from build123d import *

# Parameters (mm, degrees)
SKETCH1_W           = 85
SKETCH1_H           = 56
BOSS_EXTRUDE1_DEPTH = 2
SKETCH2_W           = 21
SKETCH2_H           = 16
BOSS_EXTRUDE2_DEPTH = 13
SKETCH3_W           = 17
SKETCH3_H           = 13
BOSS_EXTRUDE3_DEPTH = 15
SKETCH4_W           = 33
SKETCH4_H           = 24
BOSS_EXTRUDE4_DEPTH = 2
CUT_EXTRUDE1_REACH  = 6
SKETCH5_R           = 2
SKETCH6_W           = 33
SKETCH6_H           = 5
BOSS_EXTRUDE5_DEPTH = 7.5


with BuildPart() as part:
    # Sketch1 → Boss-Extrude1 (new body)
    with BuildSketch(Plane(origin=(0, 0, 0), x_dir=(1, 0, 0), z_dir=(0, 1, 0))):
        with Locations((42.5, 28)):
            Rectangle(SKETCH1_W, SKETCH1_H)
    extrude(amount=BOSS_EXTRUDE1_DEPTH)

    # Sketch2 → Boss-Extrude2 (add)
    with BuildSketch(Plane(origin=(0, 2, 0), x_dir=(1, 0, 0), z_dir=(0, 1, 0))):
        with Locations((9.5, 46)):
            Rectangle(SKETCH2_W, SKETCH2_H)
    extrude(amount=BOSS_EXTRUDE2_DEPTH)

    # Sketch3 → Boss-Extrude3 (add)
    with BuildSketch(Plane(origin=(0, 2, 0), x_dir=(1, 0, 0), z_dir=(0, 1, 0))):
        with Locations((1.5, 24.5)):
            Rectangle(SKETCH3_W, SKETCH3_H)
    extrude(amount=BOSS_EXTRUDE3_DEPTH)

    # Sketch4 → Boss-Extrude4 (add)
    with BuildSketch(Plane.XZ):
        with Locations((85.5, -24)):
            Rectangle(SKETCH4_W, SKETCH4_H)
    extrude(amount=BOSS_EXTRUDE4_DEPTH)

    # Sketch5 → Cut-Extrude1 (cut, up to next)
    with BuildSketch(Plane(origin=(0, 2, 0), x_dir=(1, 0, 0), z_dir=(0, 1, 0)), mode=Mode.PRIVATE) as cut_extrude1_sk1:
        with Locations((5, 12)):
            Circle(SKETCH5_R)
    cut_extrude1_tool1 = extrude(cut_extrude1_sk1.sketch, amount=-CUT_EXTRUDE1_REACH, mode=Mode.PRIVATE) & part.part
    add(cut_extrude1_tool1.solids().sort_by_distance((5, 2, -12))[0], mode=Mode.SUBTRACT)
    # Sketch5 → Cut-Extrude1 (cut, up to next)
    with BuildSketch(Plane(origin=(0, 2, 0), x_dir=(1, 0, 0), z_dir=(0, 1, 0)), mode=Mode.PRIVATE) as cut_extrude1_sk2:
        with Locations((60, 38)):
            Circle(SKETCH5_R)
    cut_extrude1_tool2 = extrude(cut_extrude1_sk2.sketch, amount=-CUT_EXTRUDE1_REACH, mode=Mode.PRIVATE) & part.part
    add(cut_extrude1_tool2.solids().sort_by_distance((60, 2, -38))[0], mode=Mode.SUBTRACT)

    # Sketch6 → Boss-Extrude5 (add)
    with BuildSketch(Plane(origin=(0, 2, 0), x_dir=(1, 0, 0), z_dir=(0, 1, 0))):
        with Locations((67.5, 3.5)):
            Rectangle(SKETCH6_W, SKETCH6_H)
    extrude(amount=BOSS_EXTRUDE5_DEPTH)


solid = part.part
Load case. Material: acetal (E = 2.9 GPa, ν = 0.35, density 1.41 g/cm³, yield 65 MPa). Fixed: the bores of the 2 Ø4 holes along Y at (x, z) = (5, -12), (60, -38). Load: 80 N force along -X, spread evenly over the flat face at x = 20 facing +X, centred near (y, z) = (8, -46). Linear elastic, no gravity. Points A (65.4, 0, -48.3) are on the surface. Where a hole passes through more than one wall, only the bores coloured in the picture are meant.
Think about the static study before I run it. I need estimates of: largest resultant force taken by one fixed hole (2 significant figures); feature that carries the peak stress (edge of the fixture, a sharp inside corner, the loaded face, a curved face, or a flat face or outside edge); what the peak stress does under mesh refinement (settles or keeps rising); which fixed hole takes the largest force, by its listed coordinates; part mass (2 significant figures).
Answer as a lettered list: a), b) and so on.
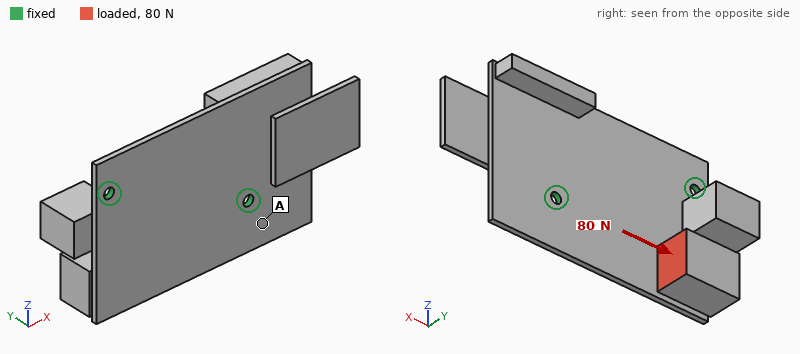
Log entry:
a) 61 N
b) edge of the fixture
c) keeps rising
d) (60, -38)
e) 28 g
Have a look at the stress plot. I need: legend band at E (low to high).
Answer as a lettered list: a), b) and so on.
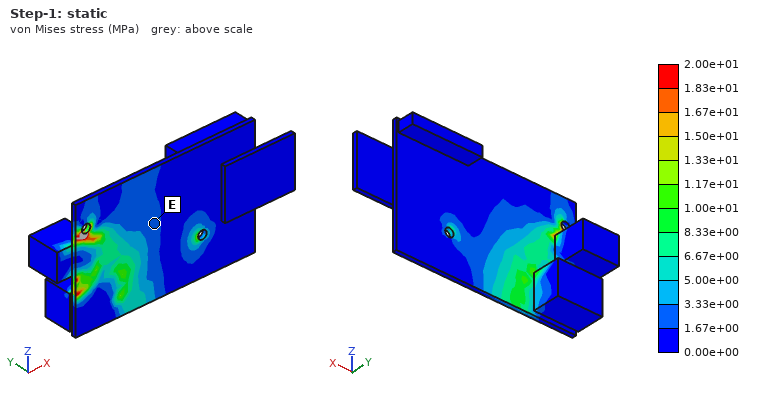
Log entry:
a) 1.67e+00 to 3.33e+00 MPa
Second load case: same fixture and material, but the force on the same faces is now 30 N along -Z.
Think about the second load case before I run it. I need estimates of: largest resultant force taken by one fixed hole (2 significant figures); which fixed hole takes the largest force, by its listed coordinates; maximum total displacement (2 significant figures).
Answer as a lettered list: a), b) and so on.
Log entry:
a) 22 N
b) (5, -12)
c) 1.1 mm
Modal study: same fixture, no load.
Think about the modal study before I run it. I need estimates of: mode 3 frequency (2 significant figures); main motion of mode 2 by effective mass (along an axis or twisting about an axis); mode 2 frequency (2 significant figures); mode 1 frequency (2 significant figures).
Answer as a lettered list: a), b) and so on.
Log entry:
a) 430 Hz
b) along Y
c) 230 Hz
d) 170 Hz
